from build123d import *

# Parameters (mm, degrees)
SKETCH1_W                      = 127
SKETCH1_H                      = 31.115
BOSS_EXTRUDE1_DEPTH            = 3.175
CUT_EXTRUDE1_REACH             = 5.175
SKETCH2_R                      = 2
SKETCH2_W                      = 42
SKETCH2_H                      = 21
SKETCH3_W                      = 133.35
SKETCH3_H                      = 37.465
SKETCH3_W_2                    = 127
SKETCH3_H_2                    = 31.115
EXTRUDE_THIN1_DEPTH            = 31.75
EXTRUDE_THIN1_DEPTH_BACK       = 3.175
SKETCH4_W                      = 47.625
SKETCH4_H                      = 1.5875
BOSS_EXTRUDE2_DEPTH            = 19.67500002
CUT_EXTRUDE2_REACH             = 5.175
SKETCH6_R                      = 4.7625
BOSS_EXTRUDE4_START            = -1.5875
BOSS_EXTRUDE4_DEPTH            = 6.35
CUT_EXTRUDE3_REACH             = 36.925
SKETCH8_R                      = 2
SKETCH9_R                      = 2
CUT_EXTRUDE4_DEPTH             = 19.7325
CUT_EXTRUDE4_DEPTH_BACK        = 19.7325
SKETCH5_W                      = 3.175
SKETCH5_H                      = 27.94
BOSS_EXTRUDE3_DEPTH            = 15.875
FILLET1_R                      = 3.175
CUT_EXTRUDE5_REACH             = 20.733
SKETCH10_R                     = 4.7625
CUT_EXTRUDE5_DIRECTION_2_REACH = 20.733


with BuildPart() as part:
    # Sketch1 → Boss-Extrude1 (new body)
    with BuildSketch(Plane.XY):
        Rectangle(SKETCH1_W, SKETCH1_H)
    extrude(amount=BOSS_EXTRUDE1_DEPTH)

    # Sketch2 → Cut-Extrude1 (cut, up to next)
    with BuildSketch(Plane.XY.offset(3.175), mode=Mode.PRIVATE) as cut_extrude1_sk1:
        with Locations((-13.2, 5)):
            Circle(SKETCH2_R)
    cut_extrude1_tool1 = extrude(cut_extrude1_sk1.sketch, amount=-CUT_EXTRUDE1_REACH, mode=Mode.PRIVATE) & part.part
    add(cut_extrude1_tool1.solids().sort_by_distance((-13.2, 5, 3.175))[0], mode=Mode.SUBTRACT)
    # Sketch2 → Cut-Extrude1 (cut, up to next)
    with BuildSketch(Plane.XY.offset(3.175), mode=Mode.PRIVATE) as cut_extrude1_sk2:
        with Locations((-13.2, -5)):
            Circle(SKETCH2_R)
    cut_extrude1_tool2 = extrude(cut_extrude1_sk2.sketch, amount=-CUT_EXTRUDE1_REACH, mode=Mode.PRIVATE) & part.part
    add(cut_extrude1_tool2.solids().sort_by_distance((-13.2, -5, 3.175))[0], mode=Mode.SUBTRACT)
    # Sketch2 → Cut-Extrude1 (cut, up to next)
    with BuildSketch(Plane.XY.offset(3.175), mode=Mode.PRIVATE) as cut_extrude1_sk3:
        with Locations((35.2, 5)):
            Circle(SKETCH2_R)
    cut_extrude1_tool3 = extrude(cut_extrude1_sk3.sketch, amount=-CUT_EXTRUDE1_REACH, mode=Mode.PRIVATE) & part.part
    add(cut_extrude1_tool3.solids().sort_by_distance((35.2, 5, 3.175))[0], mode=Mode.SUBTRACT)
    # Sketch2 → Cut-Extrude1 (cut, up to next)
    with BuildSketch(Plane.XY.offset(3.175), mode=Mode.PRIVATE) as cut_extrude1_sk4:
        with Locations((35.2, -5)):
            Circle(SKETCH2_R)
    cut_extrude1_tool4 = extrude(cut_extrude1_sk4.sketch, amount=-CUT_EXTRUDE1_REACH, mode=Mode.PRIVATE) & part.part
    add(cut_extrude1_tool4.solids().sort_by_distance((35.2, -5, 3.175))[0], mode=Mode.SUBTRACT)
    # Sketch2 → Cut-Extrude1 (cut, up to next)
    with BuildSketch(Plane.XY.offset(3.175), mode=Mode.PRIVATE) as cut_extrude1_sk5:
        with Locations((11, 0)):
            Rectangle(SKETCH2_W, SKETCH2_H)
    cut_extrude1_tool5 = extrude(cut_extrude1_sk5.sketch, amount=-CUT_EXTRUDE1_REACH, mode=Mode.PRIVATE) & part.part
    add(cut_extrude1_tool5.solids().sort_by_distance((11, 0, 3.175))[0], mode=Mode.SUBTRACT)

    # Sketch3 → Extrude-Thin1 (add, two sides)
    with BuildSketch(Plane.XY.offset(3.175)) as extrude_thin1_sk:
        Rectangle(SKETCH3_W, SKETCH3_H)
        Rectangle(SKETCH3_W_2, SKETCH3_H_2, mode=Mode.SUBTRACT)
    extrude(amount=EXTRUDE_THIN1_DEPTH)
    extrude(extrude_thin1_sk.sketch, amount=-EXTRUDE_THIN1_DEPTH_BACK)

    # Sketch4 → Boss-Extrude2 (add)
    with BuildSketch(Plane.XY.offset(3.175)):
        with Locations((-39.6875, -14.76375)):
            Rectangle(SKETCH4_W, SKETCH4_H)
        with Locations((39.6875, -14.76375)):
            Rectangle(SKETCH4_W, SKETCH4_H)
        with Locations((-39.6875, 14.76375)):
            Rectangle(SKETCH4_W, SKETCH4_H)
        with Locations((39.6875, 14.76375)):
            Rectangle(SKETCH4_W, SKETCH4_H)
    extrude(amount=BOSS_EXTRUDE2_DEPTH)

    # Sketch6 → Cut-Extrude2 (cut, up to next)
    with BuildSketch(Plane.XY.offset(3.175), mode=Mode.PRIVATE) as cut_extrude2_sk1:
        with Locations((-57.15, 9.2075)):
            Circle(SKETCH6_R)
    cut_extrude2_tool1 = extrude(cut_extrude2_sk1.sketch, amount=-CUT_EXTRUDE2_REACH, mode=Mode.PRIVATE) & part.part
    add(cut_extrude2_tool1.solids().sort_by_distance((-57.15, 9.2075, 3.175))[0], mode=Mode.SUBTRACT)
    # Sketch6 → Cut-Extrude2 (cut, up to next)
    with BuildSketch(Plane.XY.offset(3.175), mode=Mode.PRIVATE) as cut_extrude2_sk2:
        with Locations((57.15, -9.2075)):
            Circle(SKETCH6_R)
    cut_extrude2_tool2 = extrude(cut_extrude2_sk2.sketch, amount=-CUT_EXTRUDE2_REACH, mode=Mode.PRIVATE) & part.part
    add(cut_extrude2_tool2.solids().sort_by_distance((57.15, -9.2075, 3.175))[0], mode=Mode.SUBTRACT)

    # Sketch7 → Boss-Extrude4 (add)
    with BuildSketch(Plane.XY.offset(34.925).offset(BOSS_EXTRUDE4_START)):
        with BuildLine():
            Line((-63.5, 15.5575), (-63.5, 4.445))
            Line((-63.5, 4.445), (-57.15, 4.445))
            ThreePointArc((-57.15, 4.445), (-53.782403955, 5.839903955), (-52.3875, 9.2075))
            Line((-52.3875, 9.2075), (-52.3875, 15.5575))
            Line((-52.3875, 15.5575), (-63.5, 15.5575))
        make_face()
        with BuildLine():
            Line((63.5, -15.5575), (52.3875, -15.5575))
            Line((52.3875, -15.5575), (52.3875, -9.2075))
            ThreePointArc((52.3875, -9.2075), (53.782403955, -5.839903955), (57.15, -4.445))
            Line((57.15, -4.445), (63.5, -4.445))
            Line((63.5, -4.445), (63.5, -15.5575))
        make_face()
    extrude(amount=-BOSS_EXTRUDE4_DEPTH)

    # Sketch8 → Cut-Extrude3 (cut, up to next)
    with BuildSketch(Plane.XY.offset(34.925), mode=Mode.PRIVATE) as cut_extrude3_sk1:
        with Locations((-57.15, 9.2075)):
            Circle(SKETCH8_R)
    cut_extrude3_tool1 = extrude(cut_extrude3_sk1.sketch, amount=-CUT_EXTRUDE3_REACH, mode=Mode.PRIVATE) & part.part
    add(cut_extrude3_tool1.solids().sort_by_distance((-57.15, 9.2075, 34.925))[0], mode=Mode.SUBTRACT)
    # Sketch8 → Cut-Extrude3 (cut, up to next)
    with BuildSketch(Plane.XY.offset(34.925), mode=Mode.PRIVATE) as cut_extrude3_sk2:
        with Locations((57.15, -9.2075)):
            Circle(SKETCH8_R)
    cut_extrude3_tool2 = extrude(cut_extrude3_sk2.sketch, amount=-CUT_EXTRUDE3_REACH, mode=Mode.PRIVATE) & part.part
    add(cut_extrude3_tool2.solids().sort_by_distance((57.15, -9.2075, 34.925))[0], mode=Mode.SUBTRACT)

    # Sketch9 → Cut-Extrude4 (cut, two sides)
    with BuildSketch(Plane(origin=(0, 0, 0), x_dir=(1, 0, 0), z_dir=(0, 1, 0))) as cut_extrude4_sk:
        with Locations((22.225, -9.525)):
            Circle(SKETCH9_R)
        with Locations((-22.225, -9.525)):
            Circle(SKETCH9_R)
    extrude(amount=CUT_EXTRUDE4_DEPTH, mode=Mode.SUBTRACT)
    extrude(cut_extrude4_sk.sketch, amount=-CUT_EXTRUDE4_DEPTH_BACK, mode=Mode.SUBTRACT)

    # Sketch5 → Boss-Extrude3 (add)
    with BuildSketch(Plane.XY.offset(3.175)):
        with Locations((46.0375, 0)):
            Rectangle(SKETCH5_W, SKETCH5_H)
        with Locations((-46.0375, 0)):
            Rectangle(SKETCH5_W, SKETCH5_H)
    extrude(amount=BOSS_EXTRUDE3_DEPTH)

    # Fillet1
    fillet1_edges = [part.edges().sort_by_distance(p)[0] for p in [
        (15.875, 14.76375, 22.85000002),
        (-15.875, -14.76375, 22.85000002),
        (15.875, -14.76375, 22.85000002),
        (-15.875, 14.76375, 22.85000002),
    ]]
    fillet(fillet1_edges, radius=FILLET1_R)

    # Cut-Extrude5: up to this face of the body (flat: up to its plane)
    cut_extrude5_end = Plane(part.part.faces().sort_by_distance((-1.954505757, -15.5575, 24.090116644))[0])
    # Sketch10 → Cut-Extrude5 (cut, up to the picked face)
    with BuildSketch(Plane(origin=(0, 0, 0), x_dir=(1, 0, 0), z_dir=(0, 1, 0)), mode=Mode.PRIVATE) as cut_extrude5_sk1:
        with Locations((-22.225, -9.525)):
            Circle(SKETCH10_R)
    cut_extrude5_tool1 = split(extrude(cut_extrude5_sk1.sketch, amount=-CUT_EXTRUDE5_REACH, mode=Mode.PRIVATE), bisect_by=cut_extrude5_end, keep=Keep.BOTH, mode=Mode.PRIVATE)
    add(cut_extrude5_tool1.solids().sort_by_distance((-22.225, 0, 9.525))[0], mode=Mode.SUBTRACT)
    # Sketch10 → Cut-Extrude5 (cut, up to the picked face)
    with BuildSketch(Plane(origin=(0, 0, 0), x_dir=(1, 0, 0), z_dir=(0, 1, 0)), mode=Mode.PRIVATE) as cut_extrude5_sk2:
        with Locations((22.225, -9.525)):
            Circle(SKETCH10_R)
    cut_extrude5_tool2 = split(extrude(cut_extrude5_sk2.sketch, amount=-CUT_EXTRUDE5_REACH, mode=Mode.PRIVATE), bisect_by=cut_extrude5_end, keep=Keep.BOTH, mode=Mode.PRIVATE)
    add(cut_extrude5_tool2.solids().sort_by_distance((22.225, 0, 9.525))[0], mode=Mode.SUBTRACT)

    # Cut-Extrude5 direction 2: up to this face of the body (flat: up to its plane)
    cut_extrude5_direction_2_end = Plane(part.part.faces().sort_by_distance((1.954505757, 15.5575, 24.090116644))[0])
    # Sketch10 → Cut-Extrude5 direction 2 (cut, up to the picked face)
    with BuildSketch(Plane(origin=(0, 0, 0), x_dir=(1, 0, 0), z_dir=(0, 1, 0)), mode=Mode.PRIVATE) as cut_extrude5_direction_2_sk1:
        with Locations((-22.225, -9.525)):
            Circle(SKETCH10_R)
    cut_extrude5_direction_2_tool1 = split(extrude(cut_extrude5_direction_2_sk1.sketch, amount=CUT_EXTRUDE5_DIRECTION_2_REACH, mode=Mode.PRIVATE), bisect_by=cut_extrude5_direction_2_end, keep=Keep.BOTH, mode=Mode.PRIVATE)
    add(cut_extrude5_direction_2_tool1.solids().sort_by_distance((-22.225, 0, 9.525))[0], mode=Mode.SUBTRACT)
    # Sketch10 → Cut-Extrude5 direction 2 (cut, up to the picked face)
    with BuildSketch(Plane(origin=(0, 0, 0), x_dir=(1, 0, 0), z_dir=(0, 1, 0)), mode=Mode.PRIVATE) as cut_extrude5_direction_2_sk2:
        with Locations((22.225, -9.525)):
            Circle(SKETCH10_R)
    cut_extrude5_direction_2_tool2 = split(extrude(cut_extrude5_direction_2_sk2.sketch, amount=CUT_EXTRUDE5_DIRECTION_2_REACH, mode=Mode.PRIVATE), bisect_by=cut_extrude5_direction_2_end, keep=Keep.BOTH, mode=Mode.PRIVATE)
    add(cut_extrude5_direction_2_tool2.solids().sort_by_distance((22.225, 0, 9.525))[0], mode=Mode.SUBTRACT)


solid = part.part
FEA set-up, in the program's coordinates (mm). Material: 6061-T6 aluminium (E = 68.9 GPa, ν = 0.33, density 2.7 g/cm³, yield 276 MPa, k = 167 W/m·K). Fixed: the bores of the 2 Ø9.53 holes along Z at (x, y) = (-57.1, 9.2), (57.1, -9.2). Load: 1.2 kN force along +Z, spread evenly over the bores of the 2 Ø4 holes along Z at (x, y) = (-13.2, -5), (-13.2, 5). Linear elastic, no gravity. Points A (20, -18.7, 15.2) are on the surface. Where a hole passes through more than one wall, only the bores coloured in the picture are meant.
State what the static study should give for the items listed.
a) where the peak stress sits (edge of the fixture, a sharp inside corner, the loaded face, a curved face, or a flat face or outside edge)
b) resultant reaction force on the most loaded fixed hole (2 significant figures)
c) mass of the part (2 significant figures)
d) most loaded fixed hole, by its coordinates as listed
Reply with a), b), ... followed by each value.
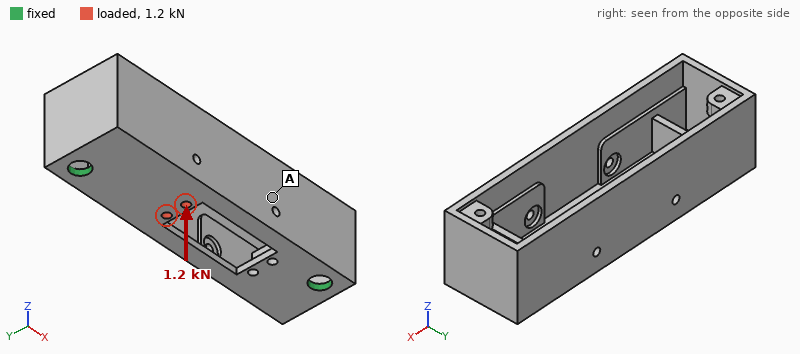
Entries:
a) the loaded face
b) 860 N
c) 150 g
d) (-57.1, 9.2)
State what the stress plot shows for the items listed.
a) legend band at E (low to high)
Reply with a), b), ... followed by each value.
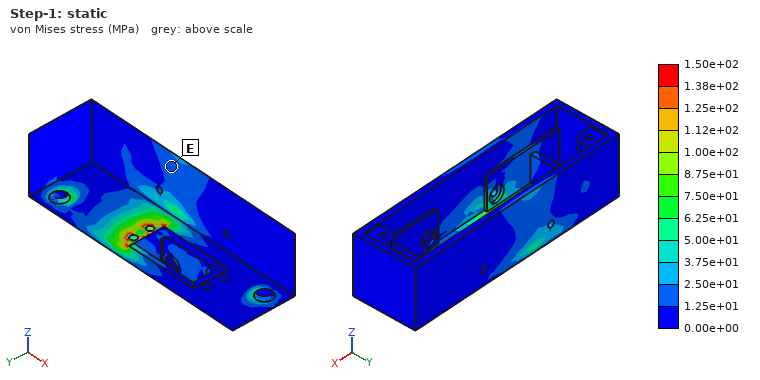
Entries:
a) 1.25e+01 to 2.50e+01 MPa
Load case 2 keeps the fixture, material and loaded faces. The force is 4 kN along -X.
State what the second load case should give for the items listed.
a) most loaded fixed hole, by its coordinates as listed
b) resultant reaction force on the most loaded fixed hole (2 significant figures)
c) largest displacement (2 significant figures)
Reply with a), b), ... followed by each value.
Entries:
a) (-57.1, 9.2)
b) 2.8 kN
c) 40 µm
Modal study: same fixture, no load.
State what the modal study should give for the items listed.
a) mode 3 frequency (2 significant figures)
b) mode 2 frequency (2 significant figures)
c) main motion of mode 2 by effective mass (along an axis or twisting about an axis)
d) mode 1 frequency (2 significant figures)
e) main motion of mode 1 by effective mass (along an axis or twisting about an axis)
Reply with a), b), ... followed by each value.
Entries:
a) 2900 Hz
b) 2600 Hz
c) along Z
d) 1900 Hz
e) along Y
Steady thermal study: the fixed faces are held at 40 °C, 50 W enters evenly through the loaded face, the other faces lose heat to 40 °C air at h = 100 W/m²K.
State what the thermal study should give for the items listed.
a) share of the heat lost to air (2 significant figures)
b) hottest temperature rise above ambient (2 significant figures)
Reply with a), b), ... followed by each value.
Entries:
a) 52 %
b) 62 K
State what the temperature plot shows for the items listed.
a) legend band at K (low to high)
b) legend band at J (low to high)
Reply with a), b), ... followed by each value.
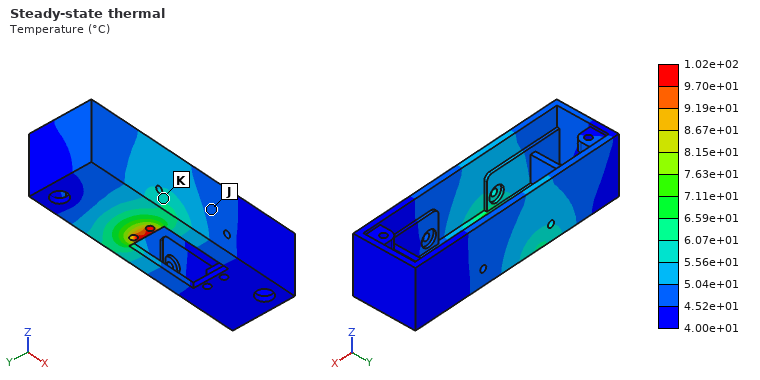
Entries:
a) 5.56e+01 to 6.07e+01 °C
b) 4.52e+01 to 5.04e+01 °C
